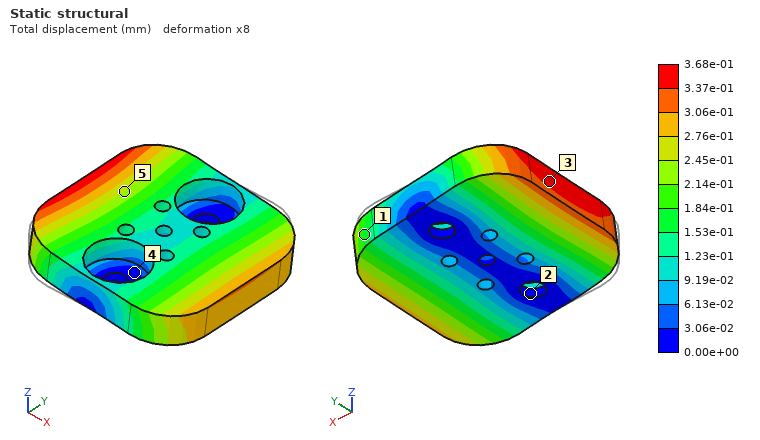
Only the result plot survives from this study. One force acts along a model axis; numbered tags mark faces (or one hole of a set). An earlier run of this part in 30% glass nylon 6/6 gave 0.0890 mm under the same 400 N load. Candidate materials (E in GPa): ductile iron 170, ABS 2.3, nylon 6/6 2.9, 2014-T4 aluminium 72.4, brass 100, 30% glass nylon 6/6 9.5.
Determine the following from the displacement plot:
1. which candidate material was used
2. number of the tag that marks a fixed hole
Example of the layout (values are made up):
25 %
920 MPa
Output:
ABS
2
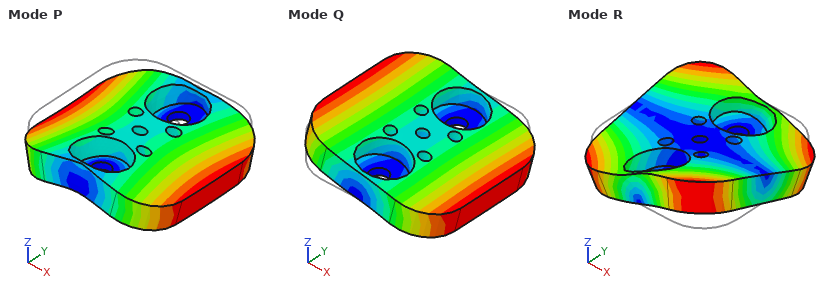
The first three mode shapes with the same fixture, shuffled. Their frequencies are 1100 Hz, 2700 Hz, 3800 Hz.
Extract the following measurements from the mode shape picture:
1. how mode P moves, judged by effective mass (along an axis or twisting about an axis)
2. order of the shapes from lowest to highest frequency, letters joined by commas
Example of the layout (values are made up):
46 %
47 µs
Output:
along Z
Q, P, R
